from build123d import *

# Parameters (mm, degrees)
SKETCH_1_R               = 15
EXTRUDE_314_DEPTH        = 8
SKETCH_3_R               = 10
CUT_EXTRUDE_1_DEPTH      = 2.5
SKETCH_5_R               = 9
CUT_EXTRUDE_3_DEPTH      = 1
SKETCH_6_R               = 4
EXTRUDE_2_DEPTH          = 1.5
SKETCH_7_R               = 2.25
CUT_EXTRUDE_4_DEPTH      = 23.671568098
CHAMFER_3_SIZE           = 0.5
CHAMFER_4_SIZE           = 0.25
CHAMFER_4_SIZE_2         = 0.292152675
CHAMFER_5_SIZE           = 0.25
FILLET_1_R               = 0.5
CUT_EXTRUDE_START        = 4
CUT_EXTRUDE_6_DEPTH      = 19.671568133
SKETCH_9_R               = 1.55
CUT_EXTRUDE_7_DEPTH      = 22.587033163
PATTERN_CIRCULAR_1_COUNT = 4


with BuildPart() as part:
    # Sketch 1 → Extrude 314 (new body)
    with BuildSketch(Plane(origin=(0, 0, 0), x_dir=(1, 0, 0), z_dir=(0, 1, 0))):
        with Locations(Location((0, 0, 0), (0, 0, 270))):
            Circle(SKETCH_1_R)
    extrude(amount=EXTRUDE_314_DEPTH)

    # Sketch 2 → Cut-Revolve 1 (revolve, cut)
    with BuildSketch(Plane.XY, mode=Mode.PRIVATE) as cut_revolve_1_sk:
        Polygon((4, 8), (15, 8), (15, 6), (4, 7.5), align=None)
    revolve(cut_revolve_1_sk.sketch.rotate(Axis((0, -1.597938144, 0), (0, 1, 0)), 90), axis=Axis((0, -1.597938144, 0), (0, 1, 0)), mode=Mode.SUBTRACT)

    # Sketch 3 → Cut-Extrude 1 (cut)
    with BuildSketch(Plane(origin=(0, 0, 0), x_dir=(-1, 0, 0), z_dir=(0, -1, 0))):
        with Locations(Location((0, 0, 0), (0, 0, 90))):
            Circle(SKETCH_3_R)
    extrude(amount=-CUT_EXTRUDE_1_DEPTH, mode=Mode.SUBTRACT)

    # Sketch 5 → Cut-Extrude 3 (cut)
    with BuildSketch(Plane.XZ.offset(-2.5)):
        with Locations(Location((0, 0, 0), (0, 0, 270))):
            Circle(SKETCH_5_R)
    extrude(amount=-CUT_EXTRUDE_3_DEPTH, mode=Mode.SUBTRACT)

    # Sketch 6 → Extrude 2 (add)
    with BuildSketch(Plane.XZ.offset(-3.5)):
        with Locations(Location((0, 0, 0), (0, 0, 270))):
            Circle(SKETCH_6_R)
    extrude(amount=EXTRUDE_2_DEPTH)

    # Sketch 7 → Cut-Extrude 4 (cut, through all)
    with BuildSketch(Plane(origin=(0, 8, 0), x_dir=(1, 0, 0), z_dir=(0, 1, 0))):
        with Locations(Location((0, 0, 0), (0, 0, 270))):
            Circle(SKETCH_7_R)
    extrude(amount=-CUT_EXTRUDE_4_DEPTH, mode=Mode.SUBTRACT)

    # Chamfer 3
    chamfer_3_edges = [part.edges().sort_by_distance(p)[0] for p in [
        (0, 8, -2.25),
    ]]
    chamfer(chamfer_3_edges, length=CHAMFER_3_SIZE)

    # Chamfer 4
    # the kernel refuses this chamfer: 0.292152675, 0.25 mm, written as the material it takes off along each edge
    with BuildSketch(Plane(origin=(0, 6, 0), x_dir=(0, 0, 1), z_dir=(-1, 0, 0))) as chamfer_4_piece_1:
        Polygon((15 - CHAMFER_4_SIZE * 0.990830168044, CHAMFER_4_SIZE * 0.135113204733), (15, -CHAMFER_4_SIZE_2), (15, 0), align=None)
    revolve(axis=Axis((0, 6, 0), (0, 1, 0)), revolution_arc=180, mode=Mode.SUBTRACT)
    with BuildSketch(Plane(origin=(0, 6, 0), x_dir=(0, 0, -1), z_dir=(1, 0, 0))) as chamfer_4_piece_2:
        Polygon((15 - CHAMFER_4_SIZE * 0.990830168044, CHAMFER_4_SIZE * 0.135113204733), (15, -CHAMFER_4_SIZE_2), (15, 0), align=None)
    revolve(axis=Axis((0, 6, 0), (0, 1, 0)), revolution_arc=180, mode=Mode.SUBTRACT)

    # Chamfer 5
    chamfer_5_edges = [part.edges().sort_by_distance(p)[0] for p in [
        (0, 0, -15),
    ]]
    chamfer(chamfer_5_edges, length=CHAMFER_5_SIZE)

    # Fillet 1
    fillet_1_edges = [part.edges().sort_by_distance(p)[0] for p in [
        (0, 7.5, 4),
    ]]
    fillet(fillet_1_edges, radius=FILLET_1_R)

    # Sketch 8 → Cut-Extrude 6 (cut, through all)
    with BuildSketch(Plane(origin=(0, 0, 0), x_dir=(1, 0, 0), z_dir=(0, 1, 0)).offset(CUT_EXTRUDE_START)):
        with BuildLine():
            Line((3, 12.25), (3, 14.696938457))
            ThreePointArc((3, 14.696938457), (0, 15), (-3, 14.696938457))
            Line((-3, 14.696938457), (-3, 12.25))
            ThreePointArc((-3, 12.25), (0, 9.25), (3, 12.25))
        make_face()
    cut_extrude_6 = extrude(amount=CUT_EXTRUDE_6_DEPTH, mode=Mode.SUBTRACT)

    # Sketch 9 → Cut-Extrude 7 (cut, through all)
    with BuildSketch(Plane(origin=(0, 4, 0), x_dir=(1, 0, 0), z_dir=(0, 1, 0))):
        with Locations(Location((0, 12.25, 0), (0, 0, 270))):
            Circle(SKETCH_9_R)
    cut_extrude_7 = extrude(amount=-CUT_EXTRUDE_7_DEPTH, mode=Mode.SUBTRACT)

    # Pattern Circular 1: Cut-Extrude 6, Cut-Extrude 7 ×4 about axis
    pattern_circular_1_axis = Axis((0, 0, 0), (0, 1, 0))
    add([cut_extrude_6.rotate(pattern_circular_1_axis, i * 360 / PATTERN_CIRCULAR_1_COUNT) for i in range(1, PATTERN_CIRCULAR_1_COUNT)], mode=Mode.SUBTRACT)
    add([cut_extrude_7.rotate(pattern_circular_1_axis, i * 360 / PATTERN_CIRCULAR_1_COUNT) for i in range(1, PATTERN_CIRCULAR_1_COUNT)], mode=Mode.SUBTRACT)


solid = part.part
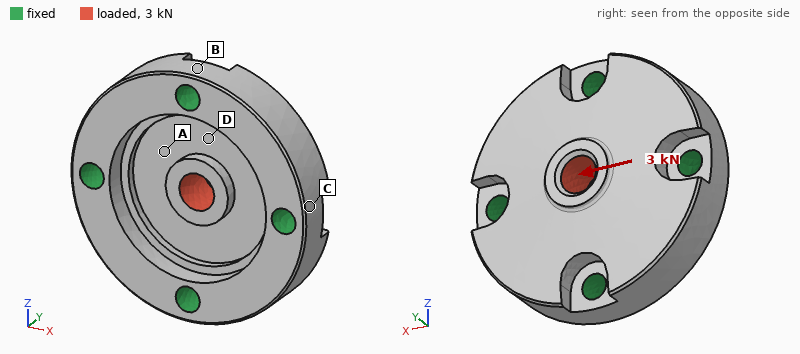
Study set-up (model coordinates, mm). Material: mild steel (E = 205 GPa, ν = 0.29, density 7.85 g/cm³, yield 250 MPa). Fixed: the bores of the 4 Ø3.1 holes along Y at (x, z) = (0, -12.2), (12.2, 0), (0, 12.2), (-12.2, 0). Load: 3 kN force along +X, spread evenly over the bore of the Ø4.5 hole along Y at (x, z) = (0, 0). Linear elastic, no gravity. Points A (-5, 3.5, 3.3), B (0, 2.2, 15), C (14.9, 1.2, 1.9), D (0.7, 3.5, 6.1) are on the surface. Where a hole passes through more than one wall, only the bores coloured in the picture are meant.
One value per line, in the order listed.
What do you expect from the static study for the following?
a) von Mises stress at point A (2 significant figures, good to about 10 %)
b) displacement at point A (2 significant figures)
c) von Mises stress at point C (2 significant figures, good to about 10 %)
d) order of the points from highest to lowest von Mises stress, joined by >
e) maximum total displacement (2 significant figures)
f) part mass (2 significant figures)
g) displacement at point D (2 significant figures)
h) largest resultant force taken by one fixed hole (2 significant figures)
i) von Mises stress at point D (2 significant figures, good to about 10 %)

55 MPa
2.3 µm
23 MPa
A > D > C > B
4.4 µm
26 g
1.8 µm
830 N
35 MPa
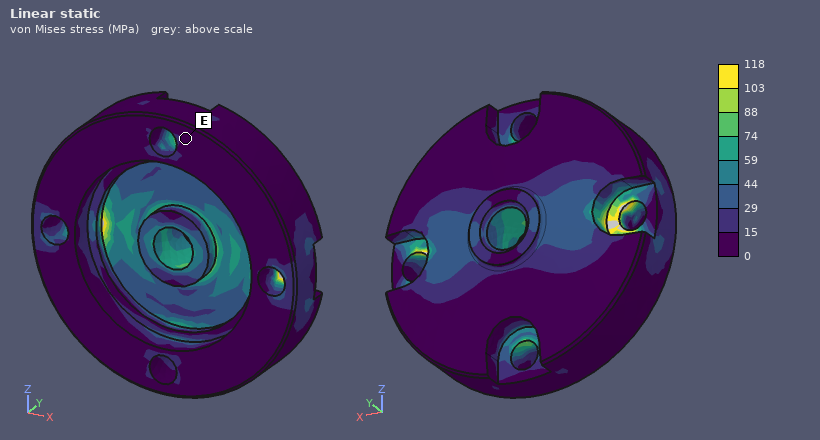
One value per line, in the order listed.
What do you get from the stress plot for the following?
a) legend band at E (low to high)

0 to 15 MPa
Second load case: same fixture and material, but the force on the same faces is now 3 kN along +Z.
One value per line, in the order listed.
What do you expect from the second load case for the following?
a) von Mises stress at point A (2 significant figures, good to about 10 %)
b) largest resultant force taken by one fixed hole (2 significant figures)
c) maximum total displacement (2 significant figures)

44 MPa
830 N
4.4 µm
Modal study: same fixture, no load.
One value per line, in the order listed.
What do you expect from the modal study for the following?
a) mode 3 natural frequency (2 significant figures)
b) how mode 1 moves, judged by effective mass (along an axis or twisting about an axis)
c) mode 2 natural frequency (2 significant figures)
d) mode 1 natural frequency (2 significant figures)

49 kHz
along Y
49 kHz
46 kHz
